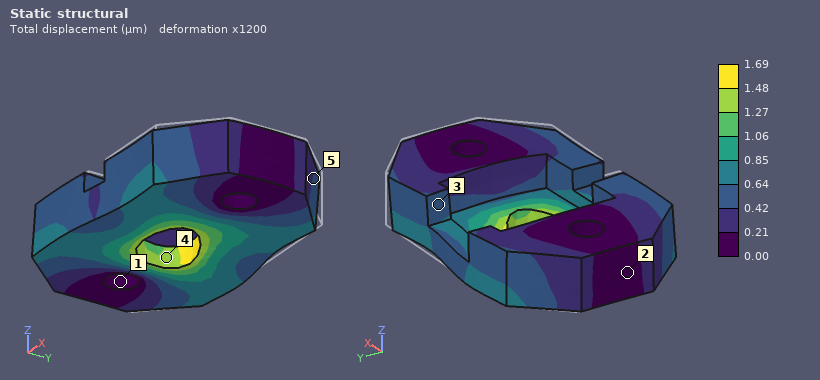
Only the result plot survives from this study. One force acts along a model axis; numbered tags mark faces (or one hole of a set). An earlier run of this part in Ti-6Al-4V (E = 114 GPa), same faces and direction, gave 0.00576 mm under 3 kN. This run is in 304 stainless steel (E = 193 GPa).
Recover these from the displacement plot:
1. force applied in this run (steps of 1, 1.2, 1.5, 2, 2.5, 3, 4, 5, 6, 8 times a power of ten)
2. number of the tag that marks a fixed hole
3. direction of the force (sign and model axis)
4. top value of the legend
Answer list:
1.5 kN
1
-X
1.69 µm
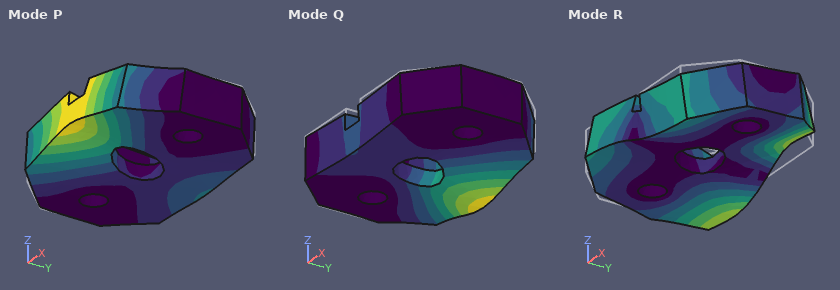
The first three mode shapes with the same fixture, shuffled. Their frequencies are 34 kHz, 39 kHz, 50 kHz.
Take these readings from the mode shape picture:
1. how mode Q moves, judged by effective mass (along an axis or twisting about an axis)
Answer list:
along Z
